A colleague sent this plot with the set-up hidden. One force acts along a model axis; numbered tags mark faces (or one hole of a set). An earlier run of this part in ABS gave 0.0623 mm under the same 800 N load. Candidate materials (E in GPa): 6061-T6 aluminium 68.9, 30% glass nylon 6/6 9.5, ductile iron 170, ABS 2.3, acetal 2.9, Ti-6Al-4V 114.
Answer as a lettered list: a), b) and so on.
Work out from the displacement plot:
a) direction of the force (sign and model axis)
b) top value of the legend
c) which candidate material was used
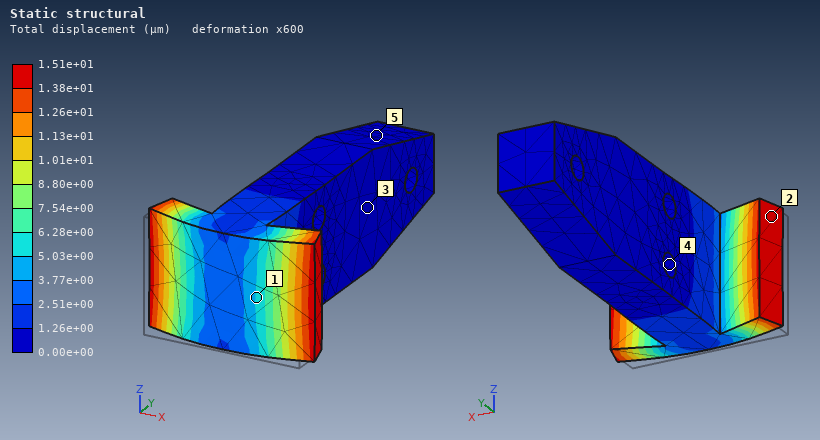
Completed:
a) +Y
b) 1.51e+01 µm
c) 30% glass nylon 6/6
